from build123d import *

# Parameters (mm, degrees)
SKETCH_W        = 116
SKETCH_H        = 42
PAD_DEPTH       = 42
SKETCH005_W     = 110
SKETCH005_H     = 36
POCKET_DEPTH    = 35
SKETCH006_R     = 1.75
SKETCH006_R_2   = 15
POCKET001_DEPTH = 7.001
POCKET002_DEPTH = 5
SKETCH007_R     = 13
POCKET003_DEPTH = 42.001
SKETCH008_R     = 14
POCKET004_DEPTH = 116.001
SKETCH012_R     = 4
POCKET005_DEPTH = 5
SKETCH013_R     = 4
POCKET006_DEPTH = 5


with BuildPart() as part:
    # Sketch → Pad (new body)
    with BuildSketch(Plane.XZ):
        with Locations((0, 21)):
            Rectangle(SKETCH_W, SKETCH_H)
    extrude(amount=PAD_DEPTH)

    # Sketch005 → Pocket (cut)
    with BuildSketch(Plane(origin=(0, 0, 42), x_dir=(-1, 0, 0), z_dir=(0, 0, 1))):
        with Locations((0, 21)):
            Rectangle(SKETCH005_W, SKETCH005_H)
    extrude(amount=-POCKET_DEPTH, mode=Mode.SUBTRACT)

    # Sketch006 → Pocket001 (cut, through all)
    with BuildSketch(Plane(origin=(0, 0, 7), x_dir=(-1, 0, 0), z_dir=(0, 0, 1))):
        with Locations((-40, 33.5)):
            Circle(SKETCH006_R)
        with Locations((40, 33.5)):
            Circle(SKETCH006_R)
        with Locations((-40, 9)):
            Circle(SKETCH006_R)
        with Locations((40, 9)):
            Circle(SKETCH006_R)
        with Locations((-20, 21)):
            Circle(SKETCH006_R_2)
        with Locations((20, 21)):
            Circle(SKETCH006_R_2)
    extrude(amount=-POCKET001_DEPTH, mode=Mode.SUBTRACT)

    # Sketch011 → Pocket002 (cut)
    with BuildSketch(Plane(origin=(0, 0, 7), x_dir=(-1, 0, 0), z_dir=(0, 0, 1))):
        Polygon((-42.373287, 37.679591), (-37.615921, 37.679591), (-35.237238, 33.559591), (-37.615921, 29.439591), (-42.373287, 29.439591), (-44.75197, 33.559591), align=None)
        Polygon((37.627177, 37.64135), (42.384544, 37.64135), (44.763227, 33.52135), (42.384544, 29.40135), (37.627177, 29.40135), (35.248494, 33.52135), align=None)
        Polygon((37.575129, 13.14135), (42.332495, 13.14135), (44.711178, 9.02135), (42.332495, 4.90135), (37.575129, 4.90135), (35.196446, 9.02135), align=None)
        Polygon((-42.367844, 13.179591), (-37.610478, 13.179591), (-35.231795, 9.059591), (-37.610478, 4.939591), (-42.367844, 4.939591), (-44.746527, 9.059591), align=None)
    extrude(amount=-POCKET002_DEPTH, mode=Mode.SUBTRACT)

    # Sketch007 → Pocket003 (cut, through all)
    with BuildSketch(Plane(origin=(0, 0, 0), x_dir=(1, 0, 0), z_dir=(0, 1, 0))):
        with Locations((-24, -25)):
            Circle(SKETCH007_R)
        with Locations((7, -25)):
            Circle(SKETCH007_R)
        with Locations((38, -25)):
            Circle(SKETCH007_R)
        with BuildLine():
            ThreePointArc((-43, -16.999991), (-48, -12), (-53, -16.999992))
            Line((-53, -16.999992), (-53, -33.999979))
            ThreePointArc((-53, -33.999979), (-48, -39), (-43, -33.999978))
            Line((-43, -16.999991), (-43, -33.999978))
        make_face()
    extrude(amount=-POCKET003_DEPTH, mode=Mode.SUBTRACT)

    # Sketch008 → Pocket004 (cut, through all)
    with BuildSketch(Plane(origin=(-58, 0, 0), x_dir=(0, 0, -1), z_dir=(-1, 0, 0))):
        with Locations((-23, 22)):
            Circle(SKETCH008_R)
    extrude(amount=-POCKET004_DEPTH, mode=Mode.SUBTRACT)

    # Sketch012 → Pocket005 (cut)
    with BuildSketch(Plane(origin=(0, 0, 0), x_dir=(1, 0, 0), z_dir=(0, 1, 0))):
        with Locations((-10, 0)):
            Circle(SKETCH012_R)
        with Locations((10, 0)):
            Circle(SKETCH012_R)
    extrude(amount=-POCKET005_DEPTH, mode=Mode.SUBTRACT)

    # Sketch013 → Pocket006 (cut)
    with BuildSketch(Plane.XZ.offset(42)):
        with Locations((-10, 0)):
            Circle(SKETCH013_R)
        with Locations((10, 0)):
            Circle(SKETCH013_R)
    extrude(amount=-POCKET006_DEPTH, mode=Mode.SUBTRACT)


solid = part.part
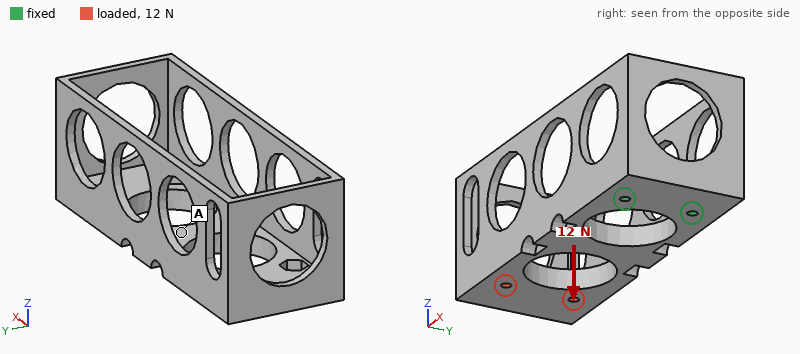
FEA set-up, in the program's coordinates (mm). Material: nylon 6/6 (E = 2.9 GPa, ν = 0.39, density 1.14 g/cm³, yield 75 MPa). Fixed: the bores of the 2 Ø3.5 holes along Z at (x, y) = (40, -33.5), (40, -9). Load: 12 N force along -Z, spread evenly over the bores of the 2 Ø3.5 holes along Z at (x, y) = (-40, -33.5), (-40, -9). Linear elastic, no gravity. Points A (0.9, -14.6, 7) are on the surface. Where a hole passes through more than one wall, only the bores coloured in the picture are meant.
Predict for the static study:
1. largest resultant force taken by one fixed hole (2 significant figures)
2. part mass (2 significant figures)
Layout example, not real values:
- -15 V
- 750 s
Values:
- 13 N
- 45 g
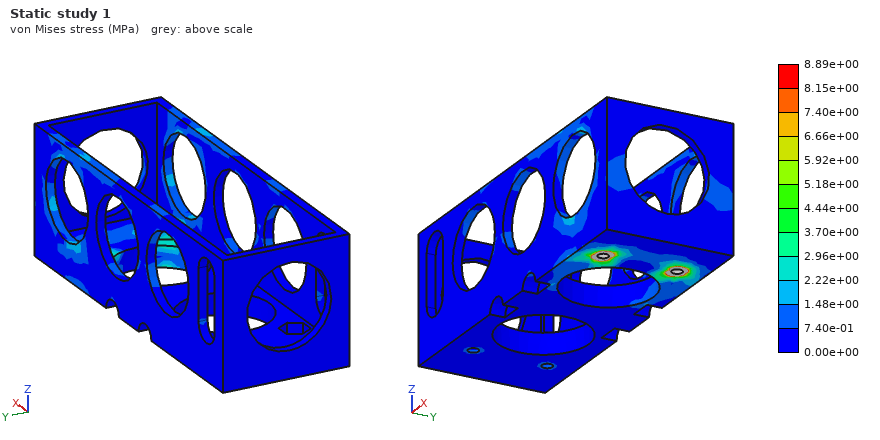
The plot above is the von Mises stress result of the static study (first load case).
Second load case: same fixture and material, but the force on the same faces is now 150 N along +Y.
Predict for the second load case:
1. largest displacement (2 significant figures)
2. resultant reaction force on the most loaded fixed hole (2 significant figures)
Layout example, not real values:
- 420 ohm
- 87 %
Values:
- 1.3 mm
- 460 N
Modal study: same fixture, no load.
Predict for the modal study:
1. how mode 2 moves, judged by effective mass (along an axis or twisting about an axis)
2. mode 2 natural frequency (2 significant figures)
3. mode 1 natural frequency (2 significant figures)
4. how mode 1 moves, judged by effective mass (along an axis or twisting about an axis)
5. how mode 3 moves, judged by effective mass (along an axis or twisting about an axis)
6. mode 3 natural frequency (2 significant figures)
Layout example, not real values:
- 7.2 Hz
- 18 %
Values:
- along Y
- 300 Hz
- 100 Hz
- along Z
- along Y
- 470 Hz
